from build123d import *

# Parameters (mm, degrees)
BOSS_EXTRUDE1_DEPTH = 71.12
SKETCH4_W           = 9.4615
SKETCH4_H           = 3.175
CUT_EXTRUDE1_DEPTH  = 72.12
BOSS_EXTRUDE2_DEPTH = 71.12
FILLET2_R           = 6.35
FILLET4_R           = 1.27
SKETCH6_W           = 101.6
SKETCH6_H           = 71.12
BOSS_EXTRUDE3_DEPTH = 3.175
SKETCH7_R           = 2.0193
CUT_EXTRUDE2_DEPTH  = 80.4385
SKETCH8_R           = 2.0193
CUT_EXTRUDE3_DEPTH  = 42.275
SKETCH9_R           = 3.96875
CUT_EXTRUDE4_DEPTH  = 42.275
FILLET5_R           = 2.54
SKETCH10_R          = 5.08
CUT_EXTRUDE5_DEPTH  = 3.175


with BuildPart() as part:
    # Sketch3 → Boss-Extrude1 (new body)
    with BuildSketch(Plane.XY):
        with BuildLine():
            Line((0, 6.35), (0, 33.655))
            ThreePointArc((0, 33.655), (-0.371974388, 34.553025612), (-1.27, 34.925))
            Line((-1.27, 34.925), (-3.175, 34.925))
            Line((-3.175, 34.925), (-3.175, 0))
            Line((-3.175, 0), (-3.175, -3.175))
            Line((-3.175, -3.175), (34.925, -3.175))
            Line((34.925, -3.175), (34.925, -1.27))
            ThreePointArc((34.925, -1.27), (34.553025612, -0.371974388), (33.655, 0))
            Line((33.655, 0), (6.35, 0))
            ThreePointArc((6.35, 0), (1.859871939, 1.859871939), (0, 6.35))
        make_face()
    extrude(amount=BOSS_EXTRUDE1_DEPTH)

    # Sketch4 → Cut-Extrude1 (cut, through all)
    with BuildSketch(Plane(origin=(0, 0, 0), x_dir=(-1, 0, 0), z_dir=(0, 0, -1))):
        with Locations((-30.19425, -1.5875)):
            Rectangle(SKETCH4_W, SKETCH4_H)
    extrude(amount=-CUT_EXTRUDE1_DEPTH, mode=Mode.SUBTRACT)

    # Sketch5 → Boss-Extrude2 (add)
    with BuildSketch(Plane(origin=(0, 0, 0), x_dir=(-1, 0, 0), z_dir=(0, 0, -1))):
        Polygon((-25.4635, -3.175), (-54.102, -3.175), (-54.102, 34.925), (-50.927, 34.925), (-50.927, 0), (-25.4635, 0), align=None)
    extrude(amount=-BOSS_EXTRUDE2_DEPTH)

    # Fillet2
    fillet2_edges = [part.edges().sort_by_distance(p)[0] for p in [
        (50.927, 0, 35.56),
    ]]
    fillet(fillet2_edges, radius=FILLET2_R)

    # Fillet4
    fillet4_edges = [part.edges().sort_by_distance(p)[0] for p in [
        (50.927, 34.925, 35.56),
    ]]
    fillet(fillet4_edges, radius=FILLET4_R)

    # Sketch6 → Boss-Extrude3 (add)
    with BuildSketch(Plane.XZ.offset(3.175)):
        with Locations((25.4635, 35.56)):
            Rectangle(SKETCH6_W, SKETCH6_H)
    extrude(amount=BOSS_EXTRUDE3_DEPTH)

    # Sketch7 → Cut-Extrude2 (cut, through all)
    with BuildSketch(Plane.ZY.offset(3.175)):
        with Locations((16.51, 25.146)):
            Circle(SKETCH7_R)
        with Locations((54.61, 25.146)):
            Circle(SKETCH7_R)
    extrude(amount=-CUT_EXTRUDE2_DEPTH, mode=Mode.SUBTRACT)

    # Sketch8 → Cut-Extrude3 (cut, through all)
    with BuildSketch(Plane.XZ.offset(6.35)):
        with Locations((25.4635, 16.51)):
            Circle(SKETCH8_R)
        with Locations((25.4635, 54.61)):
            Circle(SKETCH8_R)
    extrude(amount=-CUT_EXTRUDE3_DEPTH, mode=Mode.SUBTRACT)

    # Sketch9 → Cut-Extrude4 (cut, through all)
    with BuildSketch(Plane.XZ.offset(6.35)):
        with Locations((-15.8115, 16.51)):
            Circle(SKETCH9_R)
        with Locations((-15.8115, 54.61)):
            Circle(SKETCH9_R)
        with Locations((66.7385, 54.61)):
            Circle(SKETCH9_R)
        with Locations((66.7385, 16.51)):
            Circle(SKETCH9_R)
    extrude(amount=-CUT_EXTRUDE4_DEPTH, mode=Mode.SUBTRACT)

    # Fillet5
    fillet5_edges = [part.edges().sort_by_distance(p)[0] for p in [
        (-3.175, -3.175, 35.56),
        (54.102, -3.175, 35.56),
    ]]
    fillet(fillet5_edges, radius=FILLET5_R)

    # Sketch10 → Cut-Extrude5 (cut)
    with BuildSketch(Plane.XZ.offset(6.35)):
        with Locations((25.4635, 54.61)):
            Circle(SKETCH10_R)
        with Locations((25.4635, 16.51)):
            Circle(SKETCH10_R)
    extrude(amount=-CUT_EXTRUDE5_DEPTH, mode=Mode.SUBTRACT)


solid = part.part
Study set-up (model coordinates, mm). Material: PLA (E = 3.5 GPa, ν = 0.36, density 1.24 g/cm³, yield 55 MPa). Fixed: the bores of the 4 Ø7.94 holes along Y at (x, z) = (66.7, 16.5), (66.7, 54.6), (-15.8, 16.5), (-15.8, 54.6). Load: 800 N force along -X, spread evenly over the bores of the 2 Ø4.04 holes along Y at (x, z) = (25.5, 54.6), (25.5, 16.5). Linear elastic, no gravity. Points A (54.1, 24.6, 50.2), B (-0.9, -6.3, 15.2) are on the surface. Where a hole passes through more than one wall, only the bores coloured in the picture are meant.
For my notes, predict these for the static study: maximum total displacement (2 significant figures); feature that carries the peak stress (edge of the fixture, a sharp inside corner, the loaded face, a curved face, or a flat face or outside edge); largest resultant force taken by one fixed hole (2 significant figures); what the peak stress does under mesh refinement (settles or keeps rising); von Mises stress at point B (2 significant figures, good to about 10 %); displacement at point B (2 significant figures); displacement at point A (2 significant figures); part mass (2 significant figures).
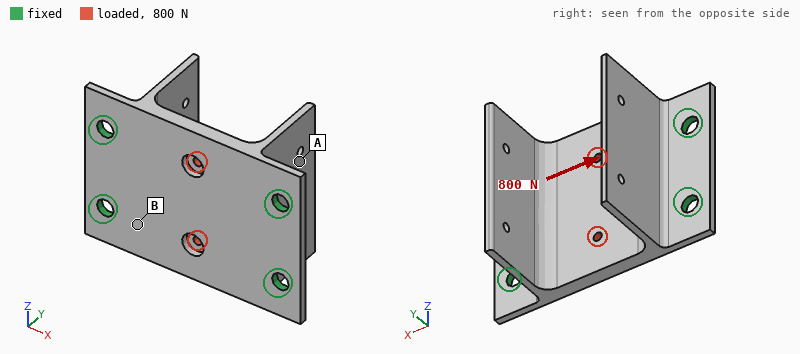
32 µm
a sharp inside corner
200 N
keeps rising
2.0 MPa
11 µm
19 µm
64 g
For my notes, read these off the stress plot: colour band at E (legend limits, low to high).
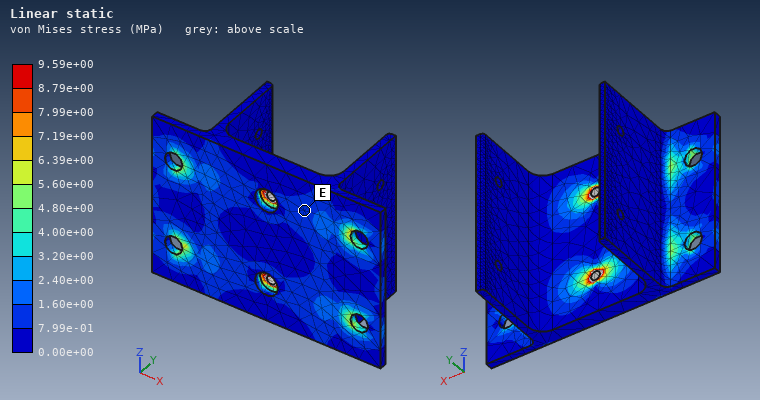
7.99e-01 to 1.60e+00 MPa
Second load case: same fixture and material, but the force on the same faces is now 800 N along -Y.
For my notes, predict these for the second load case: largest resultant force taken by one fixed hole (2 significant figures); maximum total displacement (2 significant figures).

560 N
1.0 mm
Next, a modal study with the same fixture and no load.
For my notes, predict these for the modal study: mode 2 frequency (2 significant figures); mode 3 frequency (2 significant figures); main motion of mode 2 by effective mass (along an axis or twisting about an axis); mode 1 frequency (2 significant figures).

800 Hz
990 Hz
along X
680 Hz
